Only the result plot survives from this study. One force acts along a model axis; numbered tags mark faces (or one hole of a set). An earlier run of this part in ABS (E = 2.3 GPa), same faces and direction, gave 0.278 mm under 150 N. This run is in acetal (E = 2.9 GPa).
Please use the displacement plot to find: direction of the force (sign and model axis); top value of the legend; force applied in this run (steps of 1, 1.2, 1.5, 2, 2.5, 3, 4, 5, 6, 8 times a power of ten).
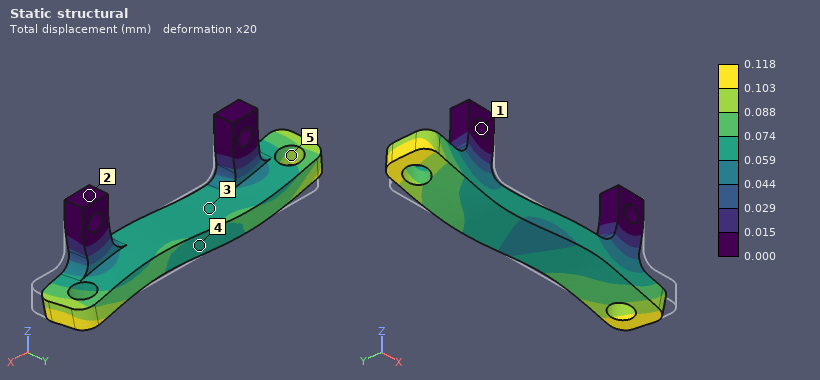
-X
0.118 mm
80 N
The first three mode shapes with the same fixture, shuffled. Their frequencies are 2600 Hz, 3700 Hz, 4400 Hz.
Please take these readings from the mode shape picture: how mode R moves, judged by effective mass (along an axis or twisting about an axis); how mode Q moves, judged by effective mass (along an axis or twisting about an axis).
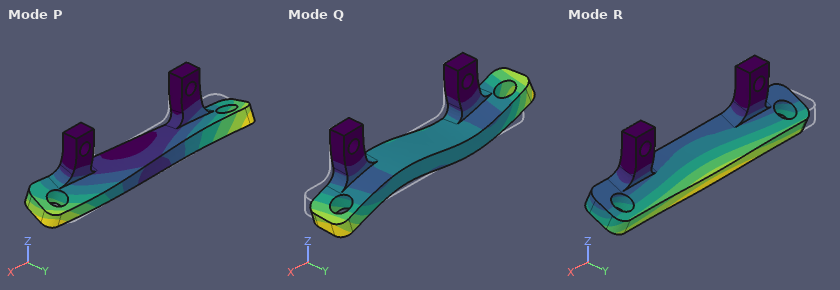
along Y
along X
